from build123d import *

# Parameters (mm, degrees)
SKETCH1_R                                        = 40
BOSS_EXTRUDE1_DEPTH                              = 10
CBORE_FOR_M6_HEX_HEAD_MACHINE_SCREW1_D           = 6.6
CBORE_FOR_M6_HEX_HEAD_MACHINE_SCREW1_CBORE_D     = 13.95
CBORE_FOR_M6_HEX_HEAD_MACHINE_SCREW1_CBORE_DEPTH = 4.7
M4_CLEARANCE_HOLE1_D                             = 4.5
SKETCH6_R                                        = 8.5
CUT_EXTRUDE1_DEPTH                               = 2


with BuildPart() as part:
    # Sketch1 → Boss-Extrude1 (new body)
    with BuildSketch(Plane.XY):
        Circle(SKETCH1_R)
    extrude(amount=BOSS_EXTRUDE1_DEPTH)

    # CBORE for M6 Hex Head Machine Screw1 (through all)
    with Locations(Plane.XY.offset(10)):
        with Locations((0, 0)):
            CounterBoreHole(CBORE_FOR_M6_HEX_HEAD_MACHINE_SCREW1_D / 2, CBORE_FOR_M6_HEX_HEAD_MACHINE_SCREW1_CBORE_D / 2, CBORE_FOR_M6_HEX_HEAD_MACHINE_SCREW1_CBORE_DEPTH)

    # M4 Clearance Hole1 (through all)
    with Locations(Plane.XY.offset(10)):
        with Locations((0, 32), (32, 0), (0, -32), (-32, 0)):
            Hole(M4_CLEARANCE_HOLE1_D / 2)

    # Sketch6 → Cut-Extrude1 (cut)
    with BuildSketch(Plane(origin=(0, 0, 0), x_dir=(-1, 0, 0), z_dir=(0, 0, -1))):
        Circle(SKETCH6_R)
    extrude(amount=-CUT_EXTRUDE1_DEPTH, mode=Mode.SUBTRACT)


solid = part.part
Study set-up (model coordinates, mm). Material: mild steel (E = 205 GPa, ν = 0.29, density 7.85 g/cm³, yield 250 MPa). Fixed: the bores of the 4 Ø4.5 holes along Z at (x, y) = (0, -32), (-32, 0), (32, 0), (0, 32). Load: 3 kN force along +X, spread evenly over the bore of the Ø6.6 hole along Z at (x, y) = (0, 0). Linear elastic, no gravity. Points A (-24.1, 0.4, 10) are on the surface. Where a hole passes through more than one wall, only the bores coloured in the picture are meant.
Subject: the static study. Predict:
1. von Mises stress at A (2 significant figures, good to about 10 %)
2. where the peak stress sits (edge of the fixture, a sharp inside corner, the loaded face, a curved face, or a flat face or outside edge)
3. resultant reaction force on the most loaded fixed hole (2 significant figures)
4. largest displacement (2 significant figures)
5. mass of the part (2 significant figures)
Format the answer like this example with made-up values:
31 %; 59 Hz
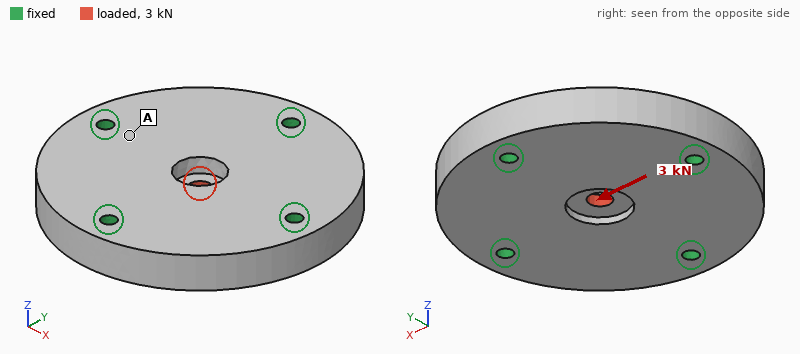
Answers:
7.6 MPa; the loaded face; 980 N; 2.0 µm; 380 g
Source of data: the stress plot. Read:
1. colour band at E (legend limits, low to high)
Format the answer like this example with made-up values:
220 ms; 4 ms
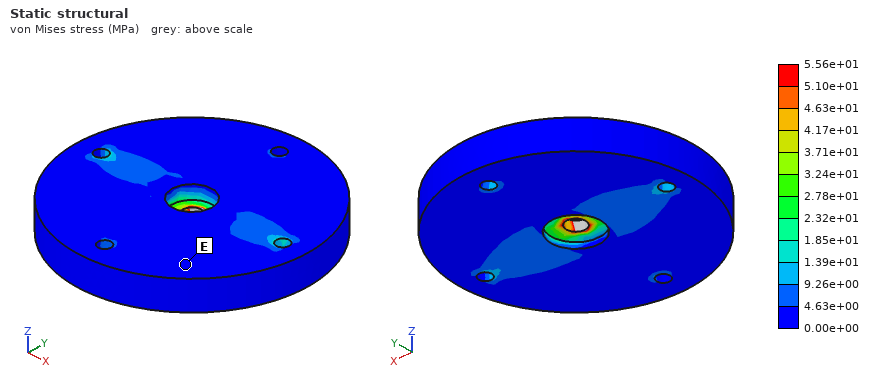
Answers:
0.00e+00 to 4.63e+00 MPa
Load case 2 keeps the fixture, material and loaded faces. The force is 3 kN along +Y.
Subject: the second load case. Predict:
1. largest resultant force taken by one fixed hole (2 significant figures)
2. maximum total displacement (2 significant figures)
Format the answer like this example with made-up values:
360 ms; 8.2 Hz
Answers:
980 N; 2.0 µm
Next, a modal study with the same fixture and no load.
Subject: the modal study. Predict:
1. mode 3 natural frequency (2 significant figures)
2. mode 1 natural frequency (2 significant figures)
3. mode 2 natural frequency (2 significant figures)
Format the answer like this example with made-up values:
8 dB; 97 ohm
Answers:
16 kHz; 14 kHz; 15 kHz
